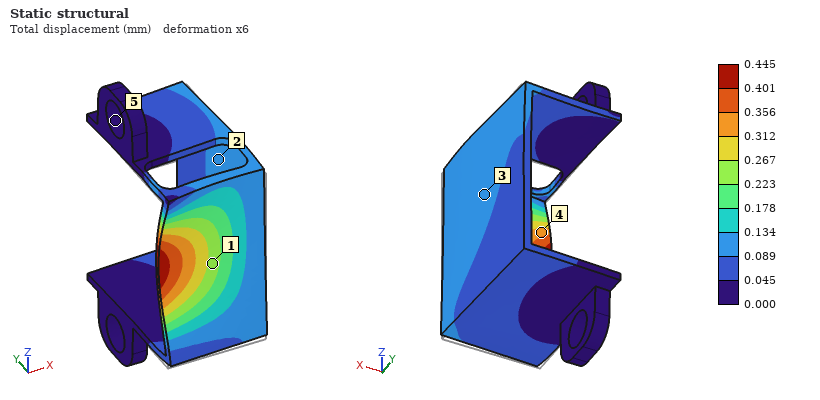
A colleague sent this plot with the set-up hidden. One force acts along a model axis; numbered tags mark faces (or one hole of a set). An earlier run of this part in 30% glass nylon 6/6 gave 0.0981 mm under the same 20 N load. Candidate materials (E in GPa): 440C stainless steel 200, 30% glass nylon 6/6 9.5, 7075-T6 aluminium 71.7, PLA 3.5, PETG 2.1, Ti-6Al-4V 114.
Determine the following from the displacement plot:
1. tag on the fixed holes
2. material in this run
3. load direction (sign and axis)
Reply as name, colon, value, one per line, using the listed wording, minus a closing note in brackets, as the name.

tag on the fixed holes: 5
material in this run: PETG
load direction: +Y
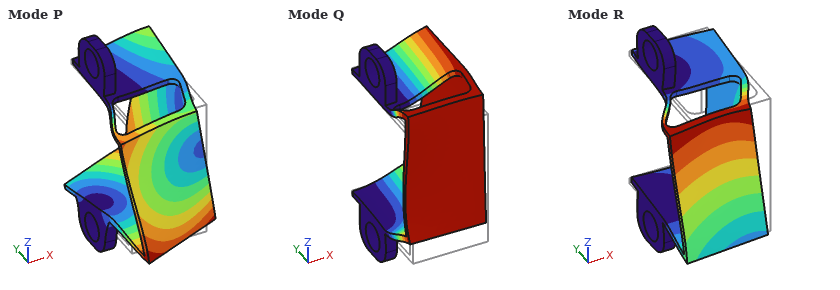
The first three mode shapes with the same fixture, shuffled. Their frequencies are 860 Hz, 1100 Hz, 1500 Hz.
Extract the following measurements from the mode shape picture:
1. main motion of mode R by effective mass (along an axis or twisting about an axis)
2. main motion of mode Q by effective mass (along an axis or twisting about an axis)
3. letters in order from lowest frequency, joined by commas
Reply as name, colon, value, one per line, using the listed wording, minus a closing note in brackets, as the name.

main motion of mode R by effective mass: along X
main motion of mode Q by effective mass: along Z
letters in order from lowest frequency, joined by commas: Q, R, P
